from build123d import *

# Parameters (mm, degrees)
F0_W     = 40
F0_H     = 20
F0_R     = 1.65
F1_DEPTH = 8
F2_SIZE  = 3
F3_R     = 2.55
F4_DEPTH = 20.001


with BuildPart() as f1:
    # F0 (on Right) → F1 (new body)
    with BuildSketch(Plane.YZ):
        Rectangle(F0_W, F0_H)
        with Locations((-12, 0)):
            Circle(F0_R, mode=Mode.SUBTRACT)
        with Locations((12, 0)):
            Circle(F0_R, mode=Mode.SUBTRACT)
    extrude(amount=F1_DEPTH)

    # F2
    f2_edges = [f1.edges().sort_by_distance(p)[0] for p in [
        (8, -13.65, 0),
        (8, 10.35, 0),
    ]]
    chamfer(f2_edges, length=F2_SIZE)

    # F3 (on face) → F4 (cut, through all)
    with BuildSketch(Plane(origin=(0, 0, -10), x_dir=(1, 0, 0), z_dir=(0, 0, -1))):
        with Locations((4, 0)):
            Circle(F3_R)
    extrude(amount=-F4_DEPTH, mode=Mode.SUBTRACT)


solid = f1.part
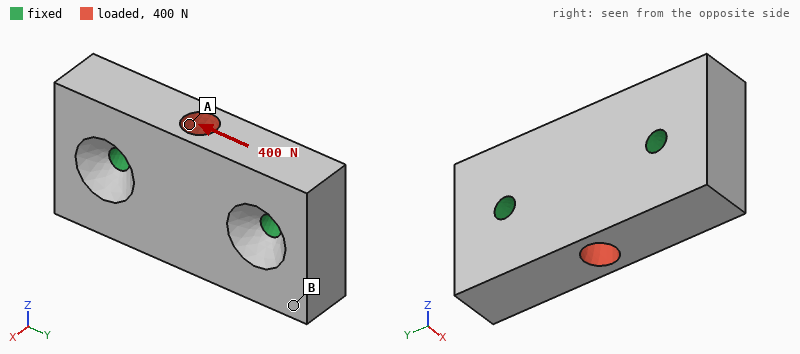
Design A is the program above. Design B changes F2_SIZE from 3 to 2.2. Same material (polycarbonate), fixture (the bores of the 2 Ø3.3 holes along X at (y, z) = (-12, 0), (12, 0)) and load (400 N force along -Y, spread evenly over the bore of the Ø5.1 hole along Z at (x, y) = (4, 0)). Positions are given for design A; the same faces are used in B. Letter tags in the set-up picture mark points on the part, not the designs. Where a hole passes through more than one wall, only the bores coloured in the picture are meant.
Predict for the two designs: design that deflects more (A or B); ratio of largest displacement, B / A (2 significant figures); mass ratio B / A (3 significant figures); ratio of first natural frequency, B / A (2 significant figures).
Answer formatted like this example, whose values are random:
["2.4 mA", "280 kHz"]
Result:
["A", "0.89", "1.01", "1.2"]
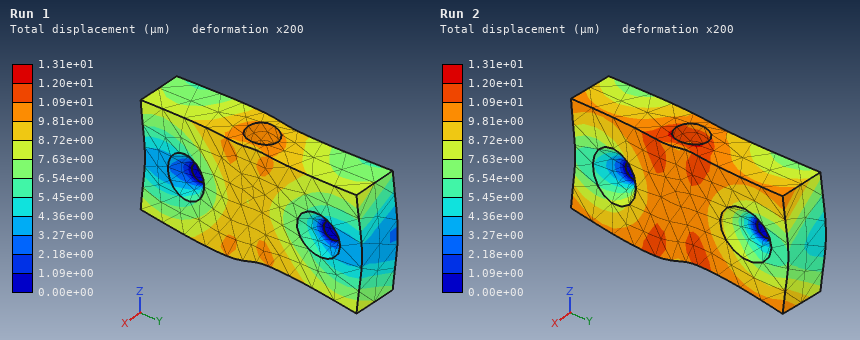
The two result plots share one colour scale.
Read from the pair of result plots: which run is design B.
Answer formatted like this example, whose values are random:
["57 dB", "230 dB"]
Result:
["Run 1"]
